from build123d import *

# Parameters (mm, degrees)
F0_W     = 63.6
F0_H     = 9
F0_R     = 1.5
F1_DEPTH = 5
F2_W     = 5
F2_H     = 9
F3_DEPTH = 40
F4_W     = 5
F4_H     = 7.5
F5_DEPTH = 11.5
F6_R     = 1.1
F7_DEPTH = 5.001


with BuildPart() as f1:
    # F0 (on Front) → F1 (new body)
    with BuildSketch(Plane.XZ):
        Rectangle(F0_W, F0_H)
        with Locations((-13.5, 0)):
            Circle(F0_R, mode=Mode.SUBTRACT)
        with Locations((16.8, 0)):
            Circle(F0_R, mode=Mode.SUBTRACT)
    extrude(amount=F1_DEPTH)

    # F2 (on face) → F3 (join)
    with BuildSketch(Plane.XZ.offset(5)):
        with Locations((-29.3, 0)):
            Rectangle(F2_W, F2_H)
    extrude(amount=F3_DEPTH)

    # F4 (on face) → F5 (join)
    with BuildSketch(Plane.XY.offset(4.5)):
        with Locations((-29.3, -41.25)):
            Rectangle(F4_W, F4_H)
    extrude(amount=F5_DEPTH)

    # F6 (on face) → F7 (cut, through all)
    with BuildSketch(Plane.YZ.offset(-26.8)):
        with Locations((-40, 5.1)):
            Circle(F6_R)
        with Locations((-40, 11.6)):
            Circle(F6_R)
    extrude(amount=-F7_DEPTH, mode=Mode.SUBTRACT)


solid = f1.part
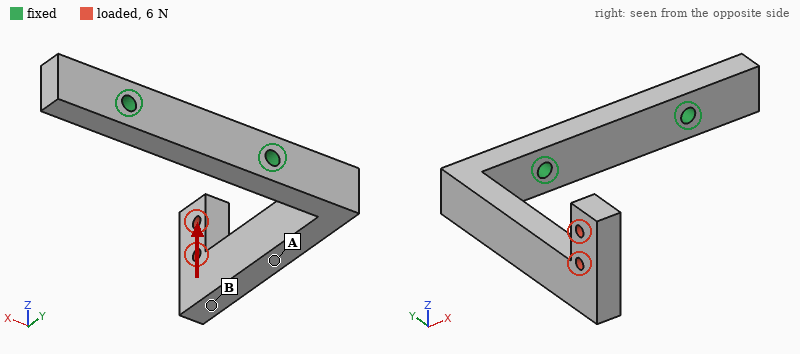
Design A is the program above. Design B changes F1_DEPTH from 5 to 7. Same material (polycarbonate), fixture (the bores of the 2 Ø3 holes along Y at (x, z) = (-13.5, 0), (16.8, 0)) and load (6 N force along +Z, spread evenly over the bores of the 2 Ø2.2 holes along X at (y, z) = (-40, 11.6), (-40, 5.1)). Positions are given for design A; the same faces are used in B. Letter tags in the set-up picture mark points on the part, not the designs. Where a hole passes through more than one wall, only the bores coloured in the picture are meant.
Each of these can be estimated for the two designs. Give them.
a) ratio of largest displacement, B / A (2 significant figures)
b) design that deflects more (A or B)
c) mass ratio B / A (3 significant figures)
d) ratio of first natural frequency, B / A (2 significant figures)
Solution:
0.56
A
1.21
1.3
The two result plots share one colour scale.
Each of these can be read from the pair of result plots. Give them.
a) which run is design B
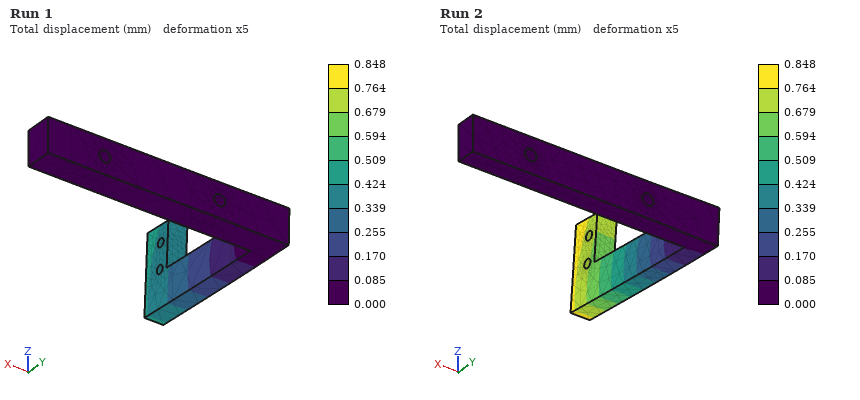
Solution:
Run 1
